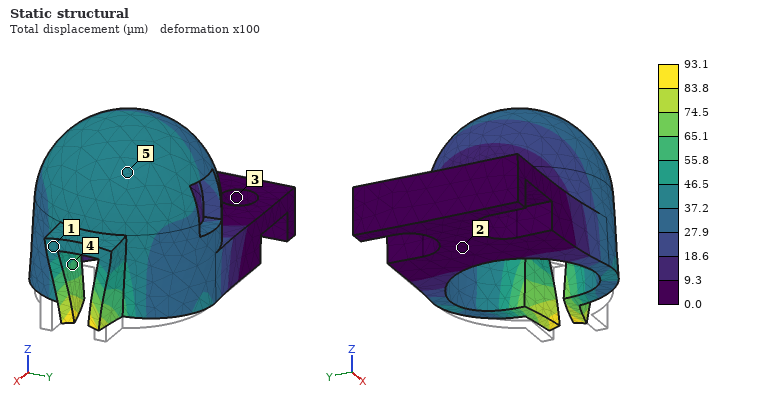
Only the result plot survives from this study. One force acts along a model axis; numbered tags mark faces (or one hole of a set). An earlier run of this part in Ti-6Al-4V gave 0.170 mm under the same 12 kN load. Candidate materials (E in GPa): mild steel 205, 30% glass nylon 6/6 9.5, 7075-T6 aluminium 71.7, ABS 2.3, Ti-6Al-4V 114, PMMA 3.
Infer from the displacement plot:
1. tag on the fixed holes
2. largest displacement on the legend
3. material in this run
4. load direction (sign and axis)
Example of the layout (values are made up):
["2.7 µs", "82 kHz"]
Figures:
["3", "93.1 µm", "mild steel", "-X"]
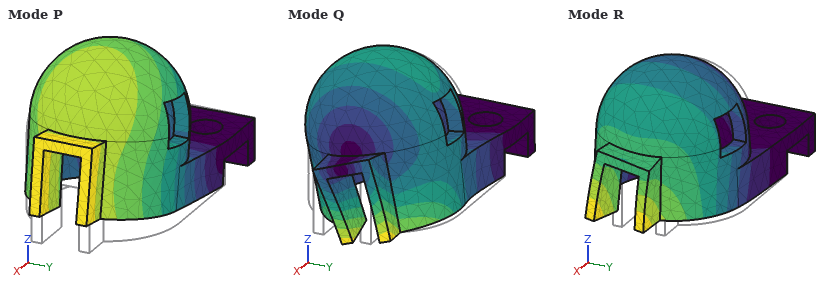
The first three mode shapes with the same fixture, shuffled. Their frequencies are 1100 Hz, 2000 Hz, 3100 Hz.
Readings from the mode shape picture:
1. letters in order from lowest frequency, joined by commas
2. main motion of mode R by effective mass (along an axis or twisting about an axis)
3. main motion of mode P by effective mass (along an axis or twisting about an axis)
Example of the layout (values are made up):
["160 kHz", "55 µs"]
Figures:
["P, R, Q", "along Y", "along Z"]
